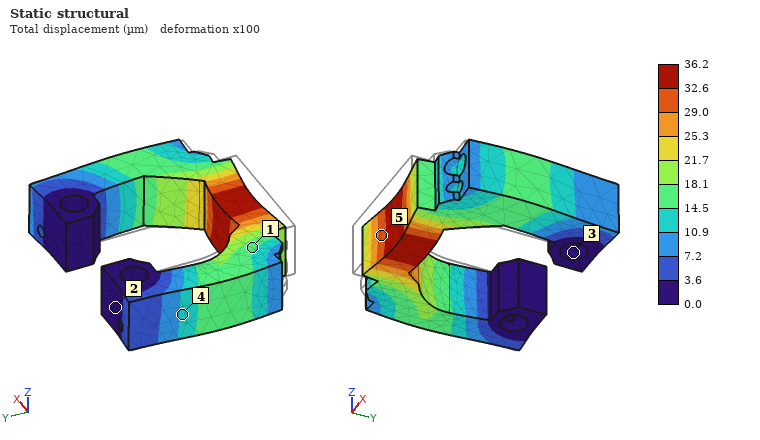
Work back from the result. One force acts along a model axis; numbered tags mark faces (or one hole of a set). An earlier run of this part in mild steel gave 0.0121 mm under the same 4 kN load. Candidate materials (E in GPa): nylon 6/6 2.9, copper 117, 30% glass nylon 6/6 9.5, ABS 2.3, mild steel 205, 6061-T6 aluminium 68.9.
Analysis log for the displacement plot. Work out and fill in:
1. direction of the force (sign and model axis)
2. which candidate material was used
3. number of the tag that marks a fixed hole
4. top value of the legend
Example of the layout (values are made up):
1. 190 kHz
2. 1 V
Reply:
1. +Y
2. 6061-T6 aluminium
3. 3
4. 36.2 µm
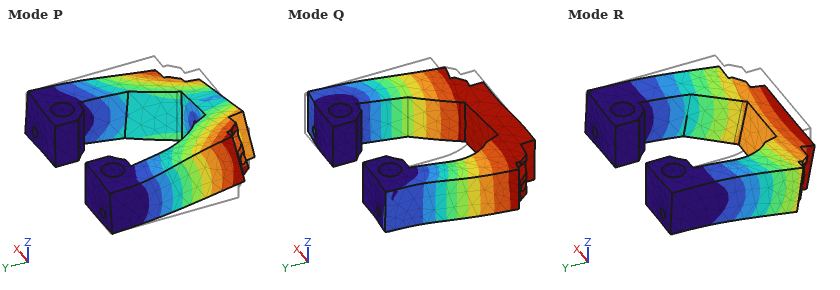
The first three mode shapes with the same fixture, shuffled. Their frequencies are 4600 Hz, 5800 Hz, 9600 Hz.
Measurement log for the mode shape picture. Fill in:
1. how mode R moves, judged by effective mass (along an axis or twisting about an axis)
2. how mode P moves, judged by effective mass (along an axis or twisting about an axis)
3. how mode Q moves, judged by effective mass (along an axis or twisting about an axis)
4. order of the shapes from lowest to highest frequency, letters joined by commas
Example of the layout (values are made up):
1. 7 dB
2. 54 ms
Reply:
1. along Z
2. twisting about Y
3. along X
4. R, Q, P
